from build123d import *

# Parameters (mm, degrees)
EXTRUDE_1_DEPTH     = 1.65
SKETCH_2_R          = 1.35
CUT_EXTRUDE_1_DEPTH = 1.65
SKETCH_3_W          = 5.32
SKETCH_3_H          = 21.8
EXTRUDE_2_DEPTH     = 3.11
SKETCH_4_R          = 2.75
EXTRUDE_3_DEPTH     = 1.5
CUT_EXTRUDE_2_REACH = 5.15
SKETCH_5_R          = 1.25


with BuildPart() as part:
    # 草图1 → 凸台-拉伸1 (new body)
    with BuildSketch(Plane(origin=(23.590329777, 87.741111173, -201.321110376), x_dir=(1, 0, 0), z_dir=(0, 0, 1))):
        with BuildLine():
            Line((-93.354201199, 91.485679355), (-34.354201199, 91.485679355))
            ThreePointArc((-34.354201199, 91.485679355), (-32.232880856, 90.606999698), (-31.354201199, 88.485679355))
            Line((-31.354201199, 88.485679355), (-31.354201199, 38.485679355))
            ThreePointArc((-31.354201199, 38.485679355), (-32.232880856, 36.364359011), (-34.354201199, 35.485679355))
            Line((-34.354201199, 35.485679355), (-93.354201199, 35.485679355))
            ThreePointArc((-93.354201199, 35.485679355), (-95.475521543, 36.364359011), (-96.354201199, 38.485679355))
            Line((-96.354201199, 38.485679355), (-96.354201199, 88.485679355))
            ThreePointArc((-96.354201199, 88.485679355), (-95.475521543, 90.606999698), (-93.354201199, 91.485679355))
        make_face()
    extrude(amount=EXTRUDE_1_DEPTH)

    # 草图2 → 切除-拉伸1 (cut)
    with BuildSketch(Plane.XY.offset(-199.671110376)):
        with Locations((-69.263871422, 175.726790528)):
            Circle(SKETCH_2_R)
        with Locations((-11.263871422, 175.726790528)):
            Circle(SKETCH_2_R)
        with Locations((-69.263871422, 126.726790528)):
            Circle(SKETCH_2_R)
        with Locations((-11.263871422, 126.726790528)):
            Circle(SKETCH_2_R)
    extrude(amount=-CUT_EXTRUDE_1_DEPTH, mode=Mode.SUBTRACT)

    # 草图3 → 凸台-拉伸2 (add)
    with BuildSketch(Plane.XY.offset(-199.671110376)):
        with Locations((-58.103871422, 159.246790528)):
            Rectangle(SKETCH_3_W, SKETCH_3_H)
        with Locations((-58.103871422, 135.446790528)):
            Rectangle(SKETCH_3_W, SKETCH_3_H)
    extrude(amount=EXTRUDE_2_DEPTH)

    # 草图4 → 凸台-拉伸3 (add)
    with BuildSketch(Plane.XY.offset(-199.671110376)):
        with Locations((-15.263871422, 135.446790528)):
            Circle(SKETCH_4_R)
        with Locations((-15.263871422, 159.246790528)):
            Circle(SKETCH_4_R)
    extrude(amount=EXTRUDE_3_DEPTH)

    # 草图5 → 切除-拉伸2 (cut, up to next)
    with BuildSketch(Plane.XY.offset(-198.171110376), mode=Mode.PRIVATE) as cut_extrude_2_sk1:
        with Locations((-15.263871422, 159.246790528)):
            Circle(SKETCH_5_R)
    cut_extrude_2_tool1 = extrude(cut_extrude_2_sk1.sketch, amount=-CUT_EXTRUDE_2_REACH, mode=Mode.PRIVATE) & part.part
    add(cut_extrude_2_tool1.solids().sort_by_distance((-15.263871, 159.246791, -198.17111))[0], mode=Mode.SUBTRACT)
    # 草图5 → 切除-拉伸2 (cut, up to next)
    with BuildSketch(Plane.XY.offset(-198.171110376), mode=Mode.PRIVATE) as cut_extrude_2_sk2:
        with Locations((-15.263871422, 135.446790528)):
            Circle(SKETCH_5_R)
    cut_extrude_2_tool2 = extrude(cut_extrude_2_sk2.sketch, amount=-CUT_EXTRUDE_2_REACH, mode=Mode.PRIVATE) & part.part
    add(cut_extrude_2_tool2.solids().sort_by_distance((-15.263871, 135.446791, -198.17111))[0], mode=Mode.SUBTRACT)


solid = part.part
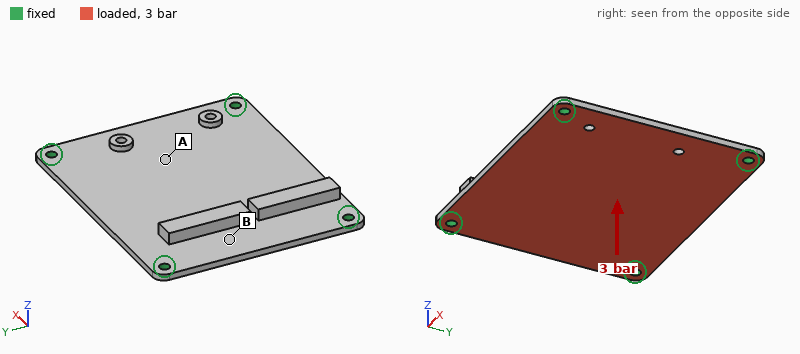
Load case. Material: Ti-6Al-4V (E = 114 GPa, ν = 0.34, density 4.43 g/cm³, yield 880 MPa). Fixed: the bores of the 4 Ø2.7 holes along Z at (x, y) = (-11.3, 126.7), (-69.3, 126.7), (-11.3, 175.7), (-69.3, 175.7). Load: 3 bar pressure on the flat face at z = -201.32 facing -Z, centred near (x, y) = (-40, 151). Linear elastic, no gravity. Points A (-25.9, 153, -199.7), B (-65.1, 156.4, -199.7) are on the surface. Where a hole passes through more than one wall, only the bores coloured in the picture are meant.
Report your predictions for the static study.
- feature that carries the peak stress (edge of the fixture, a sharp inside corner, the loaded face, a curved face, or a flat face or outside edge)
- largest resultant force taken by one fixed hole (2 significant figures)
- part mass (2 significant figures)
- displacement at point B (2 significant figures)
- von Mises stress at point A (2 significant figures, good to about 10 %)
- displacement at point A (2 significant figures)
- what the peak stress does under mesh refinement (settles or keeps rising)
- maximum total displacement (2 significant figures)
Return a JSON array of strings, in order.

["edge of the fixture", "280 N", "30 g", "0.13 mm", "84 MPa", "0.31 mm", "keeps rising", "0.39 mm"]
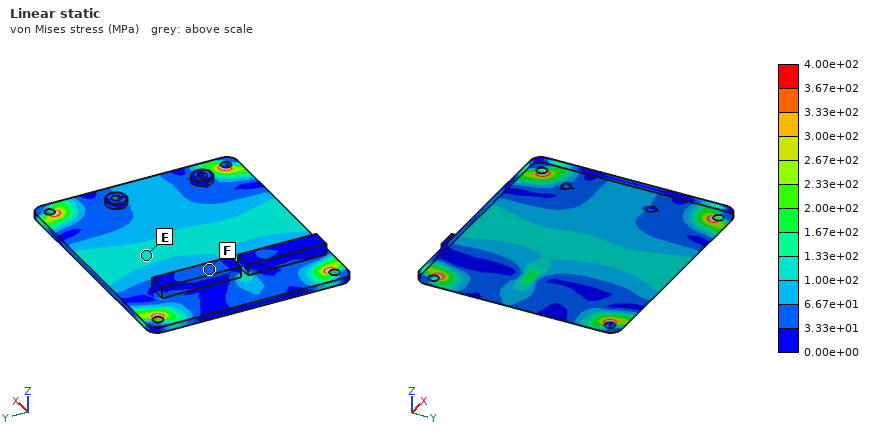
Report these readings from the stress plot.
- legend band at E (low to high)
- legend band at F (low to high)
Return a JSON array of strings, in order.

["1.00e+02 to 1.33e+02 MPa", "3.33e+01 to 6.67e+01 MPa"]
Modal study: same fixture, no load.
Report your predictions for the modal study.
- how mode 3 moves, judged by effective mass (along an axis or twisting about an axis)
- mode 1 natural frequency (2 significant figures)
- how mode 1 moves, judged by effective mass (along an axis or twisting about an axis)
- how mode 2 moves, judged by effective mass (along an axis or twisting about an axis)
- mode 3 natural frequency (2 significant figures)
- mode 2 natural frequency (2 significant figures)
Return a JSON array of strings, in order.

["twisting about Y", "1900 Hz", "along Z", "twisting about X", "3800 Hz", "3400 Hz"]
